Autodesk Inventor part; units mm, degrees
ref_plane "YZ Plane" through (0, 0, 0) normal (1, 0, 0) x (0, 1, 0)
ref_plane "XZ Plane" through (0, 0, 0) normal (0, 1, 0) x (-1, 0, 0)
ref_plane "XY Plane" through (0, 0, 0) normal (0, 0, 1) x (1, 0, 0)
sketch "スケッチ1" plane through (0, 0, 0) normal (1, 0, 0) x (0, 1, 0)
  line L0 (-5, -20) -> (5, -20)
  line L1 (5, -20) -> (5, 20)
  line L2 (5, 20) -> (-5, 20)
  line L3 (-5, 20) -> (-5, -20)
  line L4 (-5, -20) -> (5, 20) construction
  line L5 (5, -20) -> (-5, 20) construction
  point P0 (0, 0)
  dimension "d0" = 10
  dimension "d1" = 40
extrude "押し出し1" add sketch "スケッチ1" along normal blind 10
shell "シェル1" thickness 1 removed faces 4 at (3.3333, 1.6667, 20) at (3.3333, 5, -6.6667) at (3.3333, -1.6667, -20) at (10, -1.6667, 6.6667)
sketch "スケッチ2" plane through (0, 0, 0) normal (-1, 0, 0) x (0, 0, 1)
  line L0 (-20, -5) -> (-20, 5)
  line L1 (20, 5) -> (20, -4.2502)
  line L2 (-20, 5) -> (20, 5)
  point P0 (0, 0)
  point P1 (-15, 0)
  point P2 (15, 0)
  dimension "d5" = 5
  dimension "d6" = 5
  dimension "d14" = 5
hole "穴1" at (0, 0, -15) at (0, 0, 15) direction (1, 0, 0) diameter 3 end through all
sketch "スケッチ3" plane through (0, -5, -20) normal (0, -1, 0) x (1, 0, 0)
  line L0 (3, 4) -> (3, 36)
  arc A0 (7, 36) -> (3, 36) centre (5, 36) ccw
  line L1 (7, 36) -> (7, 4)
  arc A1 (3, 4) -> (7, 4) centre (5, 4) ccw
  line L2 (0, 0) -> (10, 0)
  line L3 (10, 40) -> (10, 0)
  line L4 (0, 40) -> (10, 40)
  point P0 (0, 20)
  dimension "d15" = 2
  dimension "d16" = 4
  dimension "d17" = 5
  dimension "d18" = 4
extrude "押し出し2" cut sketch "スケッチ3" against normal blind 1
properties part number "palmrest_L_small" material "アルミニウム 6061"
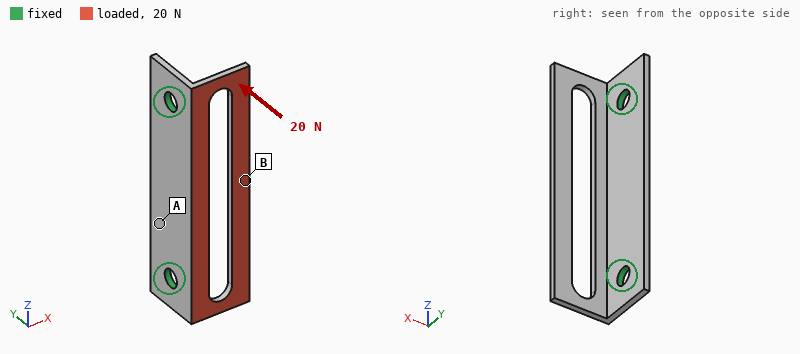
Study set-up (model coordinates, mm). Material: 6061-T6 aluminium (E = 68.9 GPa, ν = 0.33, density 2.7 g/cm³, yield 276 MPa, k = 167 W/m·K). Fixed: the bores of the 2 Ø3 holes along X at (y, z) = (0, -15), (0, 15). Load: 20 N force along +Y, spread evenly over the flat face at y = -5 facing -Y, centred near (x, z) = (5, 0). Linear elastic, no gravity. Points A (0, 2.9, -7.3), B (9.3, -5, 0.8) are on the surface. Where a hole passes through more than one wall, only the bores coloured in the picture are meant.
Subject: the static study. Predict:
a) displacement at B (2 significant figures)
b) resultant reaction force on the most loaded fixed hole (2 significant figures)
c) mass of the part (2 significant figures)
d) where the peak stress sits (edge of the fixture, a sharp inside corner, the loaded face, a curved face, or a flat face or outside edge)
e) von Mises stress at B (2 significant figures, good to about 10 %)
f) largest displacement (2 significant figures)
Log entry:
0.21 mm
10 N
1.6 g
a flat face or outside edge
39 MPa
0.22 mm
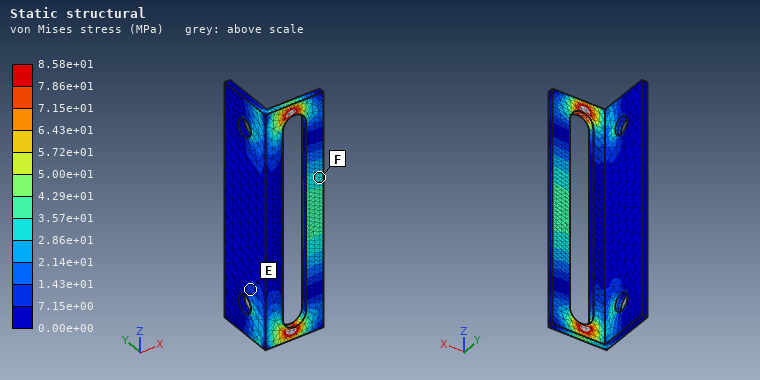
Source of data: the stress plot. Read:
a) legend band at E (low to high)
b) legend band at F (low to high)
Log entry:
7.15e+00 to 1.43e+01 MPa
2.86e+01 to 3.57e+01 MPa
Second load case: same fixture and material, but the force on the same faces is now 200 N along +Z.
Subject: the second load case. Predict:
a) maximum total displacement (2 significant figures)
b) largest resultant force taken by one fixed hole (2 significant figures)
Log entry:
74 µm
110 N
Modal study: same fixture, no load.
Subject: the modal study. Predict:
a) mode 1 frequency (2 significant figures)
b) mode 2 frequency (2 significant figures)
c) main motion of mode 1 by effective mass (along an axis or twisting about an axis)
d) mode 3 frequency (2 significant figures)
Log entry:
2200 Hz
5100 Hz
along Y
6500 Hz
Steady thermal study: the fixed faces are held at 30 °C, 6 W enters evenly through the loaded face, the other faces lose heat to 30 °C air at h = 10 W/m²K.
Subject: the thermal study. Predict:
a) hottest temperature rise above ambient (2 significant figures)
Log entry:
53 K
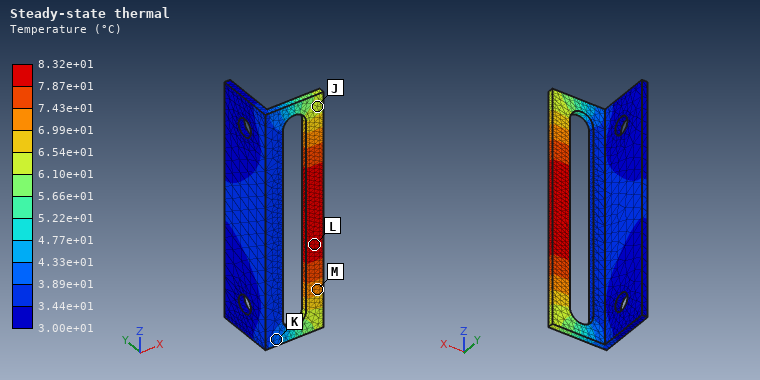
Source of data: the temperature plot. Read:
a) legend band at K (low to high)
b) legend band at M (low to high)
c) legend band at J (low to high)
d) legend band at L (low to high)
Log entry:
3.89e+01 to 4.33e+01 °C
6.99e+01 to 7.43e+01 °C
6.10e+01 to 6.54e+01 °C
7.87e+01 to 8.32e+01 °C
